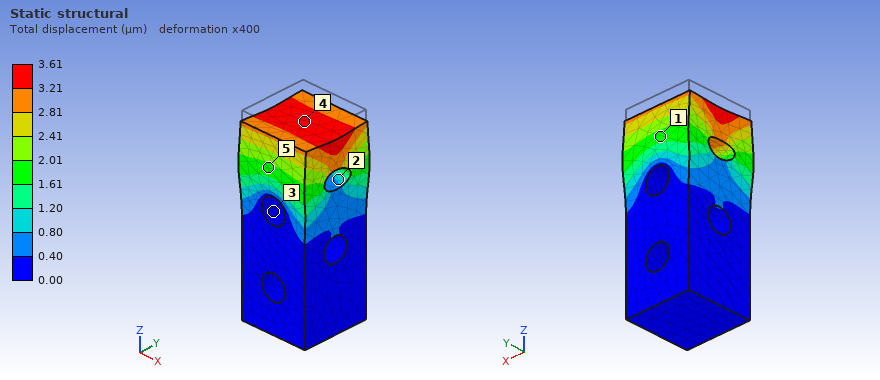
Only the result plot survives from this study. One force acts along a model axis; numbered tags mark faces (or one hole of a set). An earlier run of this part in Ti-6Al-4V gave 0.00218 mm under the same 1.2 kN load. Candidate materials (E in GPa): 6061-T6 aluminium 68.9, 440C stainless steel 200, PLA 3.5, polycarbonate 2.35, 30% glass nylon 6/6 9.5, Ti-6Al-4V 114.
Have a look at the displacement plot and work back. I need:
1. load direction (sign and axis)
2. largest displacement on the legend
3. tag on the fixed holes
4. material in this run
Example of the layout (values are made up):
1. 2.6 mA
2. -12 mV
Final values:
1. -Z
2. 3.61 µm
3. 3
4. 6061-T6 aluminium
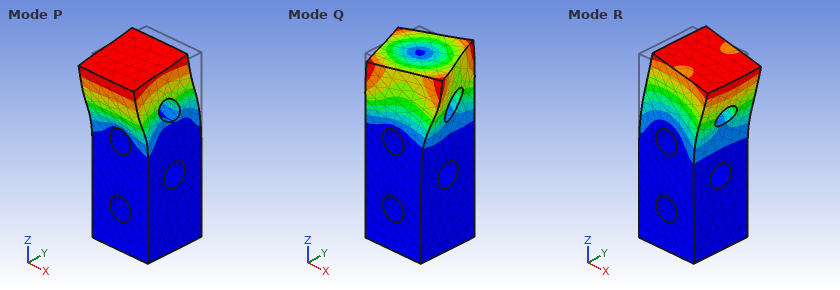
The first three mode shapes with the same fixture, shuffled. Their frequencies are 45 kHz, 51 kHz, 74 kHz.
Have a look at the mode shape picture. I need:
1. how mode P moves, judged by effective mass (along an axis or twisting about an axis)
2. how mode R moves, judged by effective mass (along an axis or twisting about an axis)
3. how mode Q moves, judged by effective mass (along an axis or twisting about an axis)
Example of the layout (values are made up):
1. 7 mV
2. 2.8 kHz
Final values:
1. along Y
2. along X
3. twisting about Z
